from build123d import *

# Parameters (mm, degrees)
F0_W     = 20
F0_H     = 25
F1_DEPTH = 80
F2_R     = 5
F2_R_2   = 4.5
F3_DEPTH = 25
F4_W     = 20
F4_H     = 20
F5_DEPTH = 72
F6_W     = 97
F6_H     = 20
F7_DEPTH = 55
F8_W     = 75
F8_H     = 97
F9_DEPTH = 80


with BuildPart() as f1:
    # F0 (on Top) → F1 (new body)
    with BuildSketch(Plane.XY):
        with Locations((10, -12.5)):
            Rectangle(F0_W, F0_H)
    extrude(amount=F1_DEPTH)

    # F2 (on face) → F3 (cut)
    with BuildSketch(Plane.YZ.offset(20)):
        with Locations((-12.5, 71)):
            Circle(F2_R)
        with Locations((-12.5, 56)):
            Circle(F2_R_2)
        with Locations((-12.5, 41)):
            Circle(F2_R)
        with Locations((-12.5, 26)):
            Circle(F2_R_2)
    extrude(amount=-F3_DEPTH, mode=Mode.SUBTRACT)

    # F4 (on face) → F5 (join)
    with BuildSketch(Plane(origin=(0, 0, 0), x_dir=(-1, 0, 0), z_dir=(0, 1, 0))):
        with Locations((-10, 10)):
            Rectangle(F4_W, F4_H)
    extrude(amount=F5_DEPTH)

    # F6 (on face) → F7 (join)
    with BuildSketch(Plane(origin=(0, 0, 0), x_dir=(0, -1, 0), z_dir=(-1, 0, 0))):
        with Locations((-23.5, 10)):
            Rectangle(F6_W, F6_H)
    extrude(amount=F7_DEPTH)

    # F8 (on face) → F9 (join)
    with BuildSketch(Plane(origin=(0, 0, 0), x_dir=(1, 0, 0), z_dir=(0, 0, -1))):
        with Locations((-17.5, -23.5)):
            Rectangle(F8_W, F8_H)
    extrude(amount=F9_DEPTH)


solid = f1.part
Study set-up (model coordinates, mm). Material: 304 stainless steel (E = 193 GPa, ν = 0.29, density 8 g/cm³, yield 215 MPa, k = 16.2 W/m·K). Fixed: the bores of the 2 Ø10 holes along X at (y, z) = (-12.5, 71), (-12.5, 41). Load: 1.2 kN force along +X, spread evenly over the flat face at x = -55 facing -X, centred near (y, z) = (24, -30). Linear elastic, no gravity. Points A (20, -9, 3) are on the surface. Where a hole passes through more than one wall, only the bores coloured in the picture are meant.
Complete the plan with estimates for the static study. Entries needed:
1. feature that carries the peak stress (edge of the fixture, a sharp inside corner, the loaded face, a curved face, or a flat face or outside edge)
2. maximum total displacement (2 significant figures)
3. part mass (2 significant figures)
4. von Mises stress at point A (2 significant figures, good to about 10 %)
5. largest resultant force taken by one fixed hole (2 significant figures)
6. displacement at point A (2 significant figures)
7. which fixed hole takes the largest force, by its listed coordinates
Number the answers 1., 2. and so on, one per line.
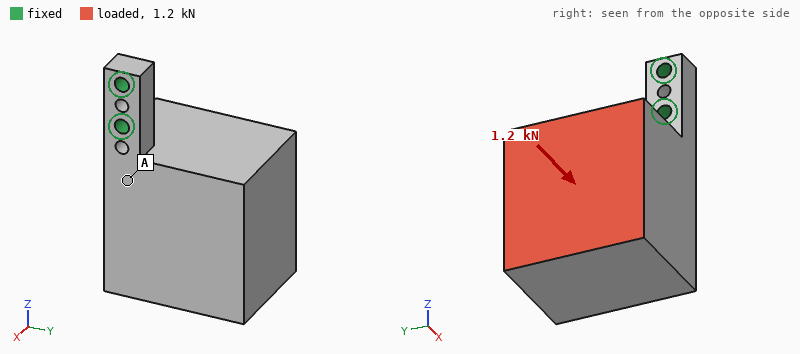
1. a curved face
2. 0.14 mm
3. 6.0 kg
4. 9.2 MPa
5. 1.5 kN
6. 0.023 mm
7. (-12.5, 41)
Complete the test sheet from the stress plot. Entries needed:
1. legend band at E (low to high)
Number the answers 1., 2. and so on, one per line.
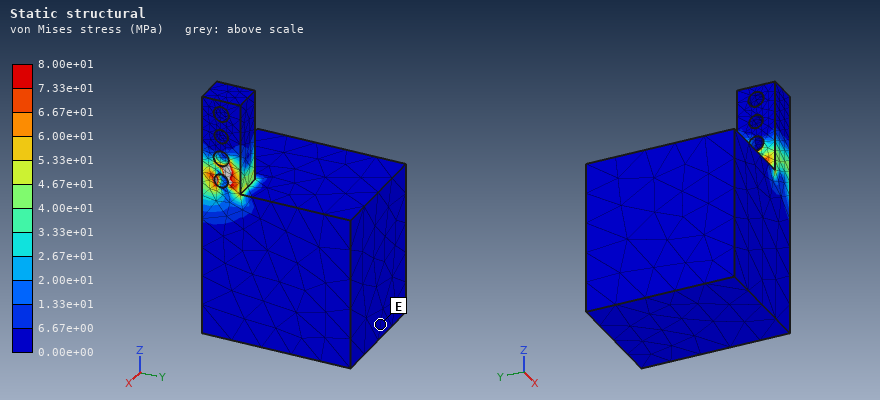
1. 0.00e+00 to 6.67e+00 MPa
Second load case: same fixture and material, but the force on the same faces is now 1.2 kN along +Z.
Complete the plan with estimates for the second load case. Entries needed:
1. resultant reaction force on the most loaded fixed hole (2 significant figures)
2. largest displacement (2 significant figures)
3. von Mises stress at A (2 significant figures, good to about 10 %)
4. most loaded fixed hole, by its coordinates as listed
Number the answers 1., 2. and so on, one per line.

1. 1.2 kN
2. 0.13 mm
3. 11 MPa
4. (-12.5, 41)
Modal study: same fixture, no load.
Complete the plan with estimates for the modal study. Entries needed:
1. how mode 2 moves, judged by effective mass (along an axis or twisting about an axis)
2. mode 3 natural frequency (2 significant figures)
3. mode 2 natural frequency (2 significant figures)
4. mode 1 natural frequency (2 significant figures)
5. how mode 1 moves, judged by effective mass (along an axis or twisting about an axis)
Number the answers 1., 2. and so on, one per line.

1. along Y
2. 540 Hz
3. 280 Hz
4. 240 Hz
5. along X
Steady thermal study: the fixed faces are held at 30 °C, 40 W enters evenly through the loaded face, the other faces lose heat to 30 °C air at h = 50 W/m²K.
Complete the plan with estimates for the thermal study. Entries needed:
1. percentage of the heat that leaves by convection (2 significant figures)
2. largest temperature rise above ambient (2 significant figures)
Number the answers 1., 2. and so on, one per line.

1. 92 %
2. 29 K
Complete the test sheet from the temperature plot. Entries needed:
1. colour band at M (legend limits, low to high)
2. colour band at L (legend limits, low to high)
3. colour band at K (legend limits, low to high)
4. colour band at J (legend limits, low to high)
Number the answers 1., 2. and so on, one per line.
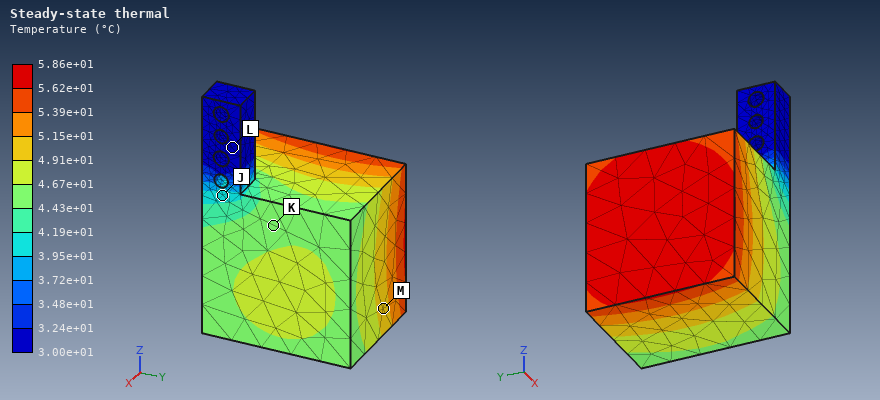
1. 4.91e+01 to 5.15e+01 °C
2. 3.00e+01 to 3.24e+01 °C
3. 4.43e+01 to 4.67e+01 °C
4. 3.95e+01 to 4.19e+01 °C
